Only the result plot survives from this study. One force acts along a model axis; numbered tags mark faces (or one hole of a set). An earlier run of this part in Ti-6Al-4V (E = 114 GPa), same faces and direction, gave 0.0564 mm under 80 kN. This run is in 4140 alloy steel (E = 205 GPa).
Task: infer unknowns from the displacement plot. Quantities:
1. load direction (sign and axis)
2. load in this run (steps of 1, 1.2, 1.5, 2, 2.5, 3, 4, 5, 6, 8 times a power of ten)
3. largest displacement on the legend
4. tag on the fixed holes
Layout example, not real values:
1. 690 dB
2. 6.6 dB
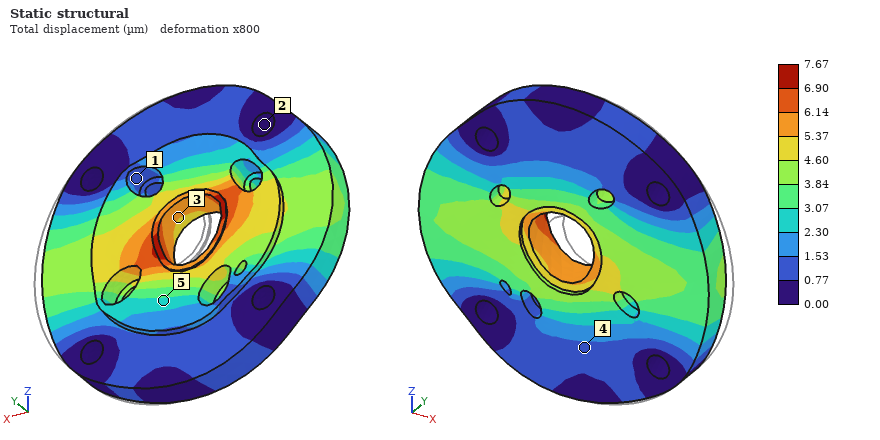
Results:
1. -X
2. 20 kN
3. 7.67 µm
4. 2
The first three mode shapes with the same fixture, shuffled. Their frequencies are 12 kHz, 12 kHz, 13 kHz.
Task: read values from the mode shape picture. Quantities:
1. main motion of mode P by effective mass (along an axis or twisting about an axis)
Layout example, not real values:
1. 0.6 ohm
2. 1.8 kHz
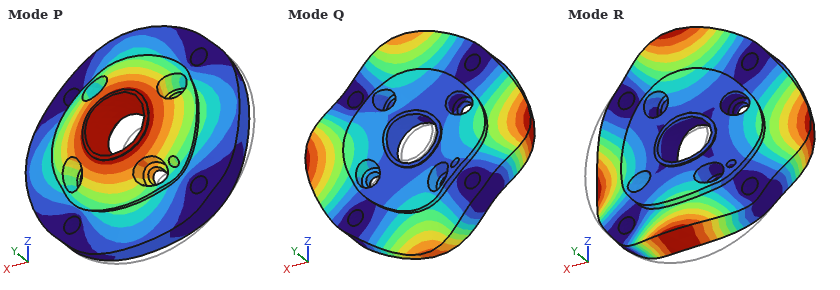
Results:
1. along Y
